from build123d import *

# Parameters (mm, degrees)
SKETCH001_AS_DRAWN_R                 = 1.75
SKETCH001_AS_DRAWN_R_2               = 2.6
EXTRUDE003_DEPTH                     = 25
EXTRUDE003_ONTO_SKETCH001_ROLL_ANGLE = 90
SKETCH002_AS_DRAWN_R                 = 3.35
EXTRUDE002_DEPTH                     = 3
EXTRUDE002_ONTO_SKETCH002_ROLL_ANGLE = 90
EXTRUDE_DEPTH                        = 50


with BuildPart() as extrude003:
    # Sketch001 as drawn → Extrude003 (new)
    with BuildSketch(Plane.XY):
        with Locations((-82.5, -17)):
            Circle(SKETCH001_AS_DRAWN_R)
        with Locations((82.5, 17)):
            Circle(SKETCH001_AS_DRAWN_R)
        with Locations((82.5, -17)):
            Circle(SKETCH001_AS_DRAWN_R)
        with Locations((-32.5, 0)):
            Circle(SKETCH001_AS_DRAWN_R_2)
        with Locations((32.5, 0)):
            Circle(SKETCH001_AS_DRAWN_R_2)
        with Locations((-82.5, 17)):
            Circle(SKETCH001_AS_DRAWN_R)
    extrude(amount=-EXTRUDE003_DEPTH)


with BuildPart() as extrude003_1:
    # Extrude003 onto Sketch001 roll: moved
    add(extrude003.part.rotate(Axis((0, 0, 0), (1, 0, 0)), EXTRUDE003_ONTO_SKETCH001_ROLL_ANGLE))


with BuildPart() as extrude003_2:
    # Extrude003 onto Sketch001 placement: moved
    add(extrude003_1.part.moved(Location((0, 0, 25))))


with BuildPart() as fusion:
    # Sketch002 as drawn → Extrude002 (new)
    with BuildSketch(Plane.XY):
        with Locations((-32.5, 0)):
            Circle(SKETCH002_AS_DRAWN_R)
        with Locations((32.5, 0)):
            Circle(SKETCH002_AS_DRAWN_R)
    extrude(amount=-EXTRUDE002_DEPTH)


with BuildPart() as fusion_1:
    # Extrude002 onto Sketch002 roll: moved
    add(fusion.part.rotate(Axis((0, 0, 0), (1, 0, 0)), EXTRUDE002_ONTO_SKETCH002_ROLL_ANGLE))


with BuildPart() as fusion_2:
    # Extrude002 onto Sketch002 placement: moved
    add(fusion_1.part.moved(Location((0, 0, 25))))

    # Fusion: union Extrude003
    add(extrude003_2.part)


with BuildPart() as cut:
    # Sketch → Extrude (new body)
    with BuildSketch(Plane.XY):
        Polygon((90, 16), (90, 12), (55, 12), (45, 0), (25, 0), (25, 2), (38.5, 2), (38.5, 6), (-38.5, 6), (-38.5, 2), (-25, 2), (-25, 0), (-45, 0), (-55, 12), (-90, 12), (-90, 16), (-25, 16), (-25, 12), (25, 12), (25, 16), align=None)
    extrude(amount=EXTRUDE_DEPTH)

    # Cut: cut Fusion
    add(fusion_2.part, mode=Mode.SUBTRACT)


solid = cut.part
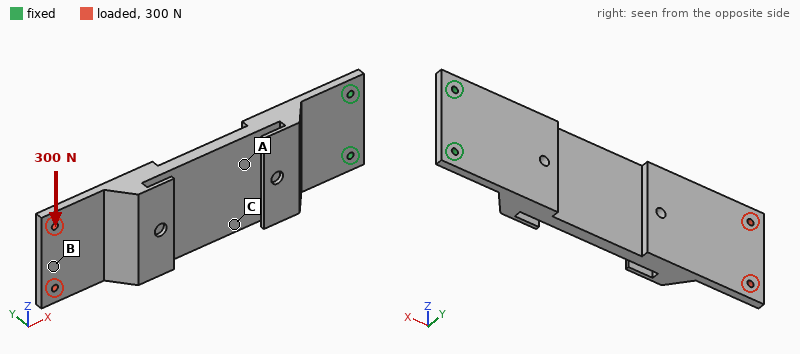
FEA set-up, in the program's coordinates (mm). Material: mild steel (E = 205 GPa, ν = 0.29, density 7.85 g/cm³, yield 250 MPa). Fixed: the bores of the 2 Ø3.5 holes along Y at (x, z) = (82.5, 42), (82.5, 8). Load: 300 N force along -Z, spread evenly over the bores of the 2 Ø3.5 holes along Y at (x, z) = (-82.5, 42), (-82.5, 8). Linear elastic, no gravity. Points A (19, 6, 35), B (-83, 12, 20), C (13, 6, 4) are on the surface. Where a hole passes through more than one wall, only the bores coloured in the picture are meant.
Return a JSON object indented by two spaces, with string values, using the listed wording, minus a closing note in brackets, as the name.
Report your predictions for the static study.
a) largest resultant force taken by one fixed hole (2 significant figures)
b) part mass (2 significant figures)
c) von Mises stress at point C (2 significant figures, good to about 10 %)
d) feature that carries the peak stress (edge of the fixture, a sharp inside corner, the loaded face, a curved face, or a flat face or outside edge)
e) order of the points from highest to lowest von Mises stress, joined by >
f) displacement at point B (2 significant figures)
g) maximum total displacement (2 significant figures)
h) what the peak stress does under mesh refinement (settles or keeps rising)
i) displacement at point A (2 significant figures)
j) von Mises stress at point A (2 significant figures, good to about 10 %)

{
  "largest resultant force taken by one fixed hole": "1.4 kN",
  "part mass": "510 g",
  "von Mises stress at point C": "9.8 MPa",
  "feature that carries the peak stress": "edge of the fixture",
  "order of the points from highest to lowest von Mises stress, joined by >": "C > A > B",
  "displacement at point B": "52 µm",
  "maximum total displacement": "59 µm",
  "what the peak stress does under mesh refinement": "keeps rising",
  "displacement at point A": "11 µm",
  "von Mises stress at point A": "5.5 MPa"
}
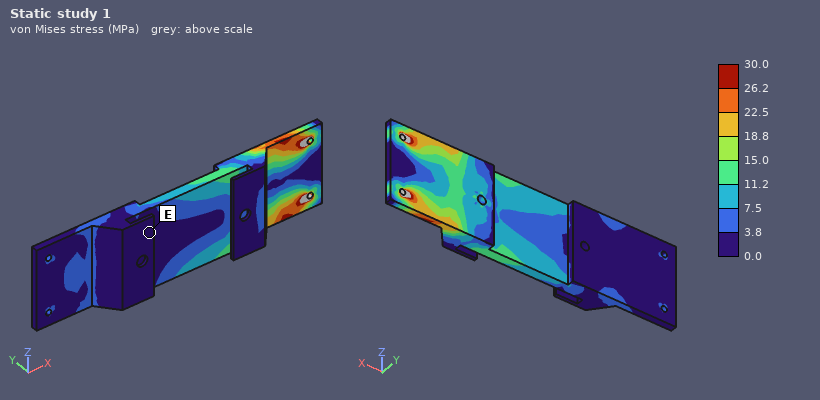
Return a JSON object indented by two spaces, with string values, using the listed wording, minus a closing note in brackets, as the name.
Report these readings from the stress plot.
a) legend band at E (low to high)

{
  "legend band at E": "0.0 to 3.8 MPa"
}
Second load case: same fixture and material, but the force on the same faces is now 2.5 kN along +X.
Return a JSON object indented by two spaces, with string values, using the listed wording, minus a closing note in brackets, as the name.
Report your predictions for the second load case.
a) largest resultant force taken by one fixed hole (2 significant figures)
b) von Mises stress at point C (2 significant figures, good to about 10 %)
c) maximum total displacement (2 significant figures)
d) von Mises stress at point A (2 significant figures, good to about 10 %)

{
  "largest resultant force taken by one fixed hole": "1.3 kN",
  "von Mises stress at point C": "34 MPa",
  "maximum total displacement": "0.37 mm",
  "von Mises stress at point A": "30 MPa"
}
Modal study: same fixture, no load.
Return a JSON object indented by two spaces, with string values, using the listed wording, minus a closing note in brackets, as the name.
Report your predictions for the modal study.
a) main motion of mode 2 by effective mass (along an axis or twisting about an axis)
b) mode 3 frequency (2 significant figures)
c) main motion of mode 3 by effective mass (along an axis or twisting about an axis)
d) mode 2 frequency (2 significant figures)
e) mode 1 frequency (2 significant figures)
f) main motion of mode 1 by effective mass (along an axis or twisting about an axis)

{
  "main motion of mode 2 by effective mass": "along Y",
  "mode 3 frequency": "1000 Hz",
  "main motion of mode 3 by effective mass": "along Z",
  "mode 2 frequency": "930 Hz",
  "mode 1 frequency": "110 Hz",
  "main motion of mode 1 by effective mass": "along Y"
}
